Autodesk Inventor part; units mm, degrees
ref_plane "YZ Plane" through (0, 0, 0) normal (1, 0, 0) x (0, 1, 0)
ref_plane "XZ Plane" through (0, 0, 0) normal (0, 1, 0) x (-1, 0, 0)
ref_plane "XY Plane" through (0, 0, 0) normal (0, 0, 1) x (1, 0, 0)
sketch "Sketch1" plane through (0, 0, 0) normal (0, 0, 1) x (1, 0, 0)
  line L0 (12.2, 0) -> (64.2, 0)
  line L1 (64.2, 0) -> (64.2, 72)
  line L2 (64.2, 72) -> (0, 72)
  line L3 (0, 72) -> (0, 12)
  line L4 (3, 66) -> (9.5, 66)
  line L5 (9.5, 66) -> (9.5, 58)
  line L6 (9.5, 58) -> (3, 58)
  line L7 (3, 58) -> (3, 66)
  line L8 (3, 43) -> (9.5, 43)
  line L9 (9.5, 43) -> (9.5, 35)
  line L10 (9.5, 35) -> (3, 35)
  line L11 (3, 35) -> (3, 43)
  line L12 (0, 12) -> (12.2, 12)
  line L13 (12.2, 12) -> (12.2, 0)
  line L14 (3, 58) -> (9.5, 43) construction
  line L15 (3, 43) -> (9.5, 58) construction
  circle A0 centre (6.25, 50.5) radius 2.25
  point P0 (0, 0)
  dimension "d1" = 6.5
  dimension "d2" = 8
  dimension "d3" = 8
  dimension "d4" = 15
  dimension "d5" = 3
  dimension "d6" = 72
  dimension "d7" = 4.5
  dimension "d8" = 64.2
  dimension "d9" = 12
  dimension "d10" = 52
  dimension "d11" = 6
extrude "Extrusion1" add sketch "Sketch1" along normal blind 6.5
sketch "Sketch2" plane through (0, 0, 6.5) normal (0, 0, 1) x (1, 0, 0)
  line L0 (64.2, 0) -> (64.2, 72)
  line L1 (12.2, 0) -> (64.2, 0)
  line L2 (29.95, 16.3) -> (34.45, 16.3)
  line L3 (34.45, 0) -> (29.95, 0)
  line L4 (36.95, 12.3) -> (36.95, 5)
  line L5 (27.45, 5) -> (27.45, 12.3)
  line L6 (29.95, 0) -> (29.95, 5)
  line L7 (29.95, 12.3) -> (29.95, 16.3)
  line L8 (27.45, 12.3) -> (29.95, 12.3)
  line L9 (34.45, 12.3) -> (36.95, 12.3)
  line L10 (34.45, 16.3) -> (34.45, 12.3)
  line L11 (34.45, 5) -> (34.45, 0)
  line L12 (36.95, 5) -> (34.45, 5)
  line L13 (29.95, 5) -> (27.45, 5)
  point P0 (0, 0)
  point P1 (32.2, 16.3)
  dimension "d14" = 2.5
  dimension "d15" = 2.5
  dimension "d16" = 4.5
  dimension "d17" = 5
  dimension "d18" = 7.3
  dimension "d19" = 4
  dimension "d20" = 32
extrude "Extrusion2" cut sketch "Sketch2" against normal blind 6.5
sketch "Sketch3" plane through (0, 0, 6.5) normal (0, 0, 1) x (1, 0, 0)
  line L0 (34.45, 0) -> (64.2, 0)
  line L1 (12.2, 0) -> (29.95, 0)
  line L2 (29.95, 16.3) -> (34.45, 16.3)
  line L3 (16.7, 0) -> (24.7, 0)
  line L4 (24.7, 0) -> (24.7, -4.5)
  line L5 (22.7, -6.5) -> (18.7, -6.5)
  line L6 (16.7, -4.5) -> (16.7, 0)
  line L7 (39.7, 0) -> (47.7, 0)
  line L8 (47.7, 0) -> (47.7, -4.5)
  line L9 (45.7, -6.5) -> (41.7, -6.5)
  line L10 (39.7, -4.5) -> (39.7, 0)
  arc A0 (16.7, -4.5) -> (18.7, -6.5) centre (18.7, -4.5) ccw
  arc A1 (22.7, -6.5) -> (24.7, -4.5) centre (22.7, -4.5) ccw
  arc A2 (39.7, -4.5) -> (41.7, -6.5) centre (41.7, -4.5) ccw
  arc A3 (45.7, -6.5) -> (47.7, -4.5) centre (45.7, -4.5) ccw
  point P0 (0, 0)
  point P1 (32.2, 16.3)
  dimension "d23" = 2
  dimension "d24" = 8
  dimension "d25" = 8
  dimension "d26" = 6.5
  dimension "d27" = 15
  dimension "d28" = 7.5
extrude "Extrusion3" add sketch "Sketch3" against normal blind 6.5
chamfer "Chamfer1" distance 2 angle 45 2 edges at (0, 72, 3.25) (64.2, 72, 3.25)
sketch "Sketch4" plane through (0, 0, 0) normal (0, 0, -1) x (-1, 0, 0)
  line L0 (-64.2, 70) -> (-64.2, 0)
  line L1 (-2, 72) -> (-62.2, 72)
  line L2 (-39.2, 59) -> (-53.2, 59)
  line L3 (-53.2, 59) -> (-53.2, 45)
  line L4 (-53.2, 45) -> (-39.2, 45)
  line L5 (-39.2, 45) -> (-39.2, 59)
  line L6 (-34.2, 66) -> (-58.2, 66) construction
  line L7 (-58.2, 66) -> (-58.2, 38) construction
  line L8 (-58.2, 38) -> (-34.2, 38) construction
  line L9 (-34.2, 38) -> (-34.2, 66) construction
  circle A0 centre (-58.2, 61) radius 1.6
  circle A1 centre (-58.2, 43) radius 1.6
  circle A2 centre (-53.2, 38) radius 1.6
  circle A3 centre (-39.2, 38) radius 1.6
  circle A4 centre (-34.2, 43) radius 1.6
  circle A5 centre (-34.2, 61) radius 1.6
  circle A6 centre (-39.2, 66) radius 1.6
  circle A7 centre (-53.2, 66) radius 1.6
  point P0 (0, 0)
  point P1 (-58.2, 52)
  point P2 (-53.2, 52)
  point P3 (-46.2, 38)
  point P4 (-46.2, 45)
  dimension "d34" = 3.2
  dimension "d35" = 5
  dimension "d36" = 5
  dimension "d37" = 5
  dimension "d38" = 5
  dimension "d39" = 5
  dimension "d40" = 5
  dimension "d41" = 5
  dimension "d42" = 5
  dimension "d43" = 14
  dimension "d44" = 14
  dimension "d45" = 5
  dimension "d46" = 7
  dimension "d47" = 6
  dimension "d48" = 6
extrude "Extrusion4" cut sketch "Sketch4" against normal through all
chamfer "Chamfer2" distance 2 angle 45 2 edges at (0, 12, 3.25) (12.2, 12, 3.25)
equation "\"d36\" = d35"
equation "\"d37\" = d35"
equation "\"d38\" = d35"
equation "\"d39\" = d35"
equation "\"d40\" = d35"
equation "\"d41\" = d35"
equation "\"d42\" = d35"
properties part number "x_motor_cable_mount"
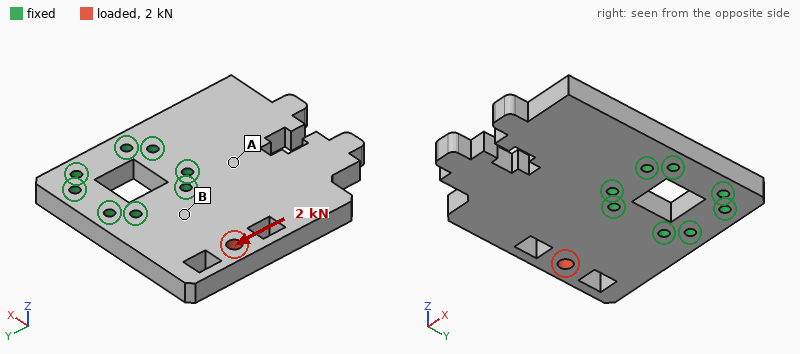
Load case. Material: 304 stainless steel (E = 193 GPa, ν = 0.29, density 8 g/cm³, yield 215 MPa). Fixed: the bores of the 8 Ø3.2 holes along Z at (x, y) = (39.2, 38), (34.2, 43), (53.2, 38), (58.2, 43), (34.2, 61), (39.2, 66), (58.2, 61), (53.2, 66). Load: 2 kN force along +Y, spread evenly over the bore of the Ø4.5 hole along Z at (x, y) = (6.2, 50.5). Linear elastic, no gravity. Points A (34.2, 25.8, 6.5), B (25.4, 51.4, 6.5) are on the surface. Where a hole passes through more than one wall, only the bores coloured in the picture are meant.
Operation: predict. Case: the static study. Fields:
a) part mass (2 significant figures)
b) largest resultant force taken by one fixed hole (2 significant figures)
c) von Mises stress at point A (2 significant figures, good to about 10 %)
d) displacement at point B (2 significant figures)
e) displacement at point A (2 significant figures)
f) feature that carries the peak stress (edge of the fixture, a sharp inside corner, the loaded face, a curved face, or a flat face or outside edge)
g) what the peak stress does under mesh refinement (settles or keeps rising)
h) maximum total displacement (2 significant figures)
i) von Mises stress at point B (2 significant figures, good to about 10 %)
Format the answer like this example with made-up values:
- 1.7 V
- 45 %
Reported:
- 210 g
- 1.3 kN
- 6.1 MPa
- 1.3 µm
- 1.7 µm
- edge of the fixture
- keeps rising
- 7.1 µm
- 16 MPa
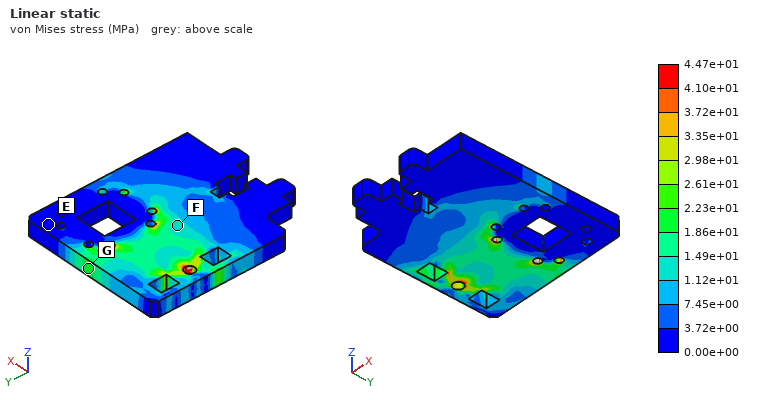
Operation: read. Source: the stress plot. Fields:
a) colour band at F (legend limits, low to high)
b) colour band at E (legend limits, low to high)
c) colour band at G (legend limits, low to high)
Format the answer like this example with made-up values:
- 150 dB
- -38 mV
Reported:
- 1.12e+01 to 1.49e+01 MPa
- 0.00e+00 to 3.72e+00 MPa
- 1.86e+01 to 2.23e+01 MPa
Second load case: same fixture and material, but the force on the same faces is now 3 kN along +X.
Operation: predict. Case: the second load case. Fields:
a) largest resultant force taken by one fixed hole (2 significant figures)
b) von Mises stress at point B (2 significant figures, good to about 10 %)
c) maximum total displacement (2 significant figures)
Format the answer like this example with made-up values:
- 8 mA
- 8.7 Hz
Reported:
- 1.1 kN
- 14 MPa
- 4.4 µm
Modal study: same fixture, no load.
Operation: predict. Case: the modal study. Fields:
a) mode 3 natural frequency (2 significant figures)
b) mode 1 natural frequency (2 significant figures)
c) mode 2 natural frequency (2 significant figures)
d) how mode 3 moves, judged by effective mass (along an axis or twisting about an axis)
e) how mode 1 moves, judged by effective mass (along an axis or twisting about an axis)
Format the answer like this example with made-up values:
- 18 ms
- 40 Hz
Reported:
- 5000 Hz
- 2700 Hz
- 3700 Hz
- along Z
- along Z
